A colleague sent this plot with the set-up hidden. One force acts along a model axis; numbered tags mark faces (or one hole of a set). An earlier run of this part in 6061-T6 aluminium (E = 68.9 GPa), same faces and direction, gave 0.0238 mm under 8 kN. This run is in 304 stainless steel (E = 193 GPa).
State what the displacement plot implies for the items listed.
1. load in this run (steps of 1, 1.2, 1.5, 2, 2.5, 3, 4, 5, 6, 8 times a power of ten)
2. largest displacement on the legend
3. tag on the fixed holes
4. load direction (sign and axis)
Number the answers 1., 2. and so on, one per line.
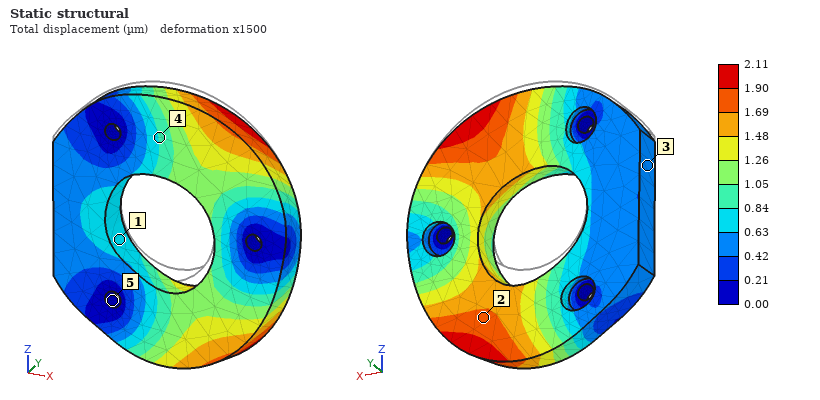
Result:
1. 2 kN
2. 2.11 µm
3. 5
4. -Z
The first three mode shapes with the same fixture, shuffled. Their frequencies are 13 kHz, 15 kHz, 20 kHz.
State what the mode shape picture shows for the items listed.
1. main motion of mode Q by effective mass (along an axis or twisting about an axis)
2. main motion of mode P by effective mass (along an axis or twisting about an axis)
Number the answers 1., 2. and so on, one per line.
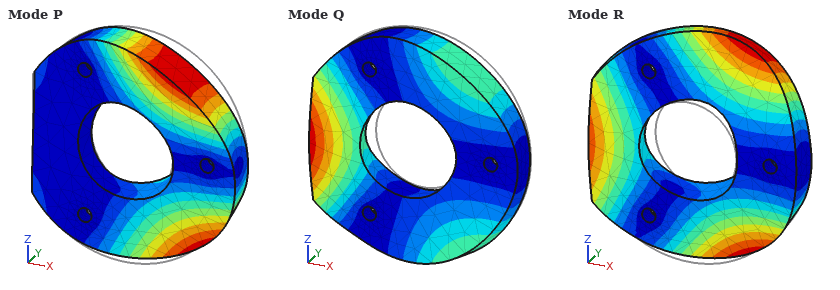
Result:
1. along Y
2. twisting about X
